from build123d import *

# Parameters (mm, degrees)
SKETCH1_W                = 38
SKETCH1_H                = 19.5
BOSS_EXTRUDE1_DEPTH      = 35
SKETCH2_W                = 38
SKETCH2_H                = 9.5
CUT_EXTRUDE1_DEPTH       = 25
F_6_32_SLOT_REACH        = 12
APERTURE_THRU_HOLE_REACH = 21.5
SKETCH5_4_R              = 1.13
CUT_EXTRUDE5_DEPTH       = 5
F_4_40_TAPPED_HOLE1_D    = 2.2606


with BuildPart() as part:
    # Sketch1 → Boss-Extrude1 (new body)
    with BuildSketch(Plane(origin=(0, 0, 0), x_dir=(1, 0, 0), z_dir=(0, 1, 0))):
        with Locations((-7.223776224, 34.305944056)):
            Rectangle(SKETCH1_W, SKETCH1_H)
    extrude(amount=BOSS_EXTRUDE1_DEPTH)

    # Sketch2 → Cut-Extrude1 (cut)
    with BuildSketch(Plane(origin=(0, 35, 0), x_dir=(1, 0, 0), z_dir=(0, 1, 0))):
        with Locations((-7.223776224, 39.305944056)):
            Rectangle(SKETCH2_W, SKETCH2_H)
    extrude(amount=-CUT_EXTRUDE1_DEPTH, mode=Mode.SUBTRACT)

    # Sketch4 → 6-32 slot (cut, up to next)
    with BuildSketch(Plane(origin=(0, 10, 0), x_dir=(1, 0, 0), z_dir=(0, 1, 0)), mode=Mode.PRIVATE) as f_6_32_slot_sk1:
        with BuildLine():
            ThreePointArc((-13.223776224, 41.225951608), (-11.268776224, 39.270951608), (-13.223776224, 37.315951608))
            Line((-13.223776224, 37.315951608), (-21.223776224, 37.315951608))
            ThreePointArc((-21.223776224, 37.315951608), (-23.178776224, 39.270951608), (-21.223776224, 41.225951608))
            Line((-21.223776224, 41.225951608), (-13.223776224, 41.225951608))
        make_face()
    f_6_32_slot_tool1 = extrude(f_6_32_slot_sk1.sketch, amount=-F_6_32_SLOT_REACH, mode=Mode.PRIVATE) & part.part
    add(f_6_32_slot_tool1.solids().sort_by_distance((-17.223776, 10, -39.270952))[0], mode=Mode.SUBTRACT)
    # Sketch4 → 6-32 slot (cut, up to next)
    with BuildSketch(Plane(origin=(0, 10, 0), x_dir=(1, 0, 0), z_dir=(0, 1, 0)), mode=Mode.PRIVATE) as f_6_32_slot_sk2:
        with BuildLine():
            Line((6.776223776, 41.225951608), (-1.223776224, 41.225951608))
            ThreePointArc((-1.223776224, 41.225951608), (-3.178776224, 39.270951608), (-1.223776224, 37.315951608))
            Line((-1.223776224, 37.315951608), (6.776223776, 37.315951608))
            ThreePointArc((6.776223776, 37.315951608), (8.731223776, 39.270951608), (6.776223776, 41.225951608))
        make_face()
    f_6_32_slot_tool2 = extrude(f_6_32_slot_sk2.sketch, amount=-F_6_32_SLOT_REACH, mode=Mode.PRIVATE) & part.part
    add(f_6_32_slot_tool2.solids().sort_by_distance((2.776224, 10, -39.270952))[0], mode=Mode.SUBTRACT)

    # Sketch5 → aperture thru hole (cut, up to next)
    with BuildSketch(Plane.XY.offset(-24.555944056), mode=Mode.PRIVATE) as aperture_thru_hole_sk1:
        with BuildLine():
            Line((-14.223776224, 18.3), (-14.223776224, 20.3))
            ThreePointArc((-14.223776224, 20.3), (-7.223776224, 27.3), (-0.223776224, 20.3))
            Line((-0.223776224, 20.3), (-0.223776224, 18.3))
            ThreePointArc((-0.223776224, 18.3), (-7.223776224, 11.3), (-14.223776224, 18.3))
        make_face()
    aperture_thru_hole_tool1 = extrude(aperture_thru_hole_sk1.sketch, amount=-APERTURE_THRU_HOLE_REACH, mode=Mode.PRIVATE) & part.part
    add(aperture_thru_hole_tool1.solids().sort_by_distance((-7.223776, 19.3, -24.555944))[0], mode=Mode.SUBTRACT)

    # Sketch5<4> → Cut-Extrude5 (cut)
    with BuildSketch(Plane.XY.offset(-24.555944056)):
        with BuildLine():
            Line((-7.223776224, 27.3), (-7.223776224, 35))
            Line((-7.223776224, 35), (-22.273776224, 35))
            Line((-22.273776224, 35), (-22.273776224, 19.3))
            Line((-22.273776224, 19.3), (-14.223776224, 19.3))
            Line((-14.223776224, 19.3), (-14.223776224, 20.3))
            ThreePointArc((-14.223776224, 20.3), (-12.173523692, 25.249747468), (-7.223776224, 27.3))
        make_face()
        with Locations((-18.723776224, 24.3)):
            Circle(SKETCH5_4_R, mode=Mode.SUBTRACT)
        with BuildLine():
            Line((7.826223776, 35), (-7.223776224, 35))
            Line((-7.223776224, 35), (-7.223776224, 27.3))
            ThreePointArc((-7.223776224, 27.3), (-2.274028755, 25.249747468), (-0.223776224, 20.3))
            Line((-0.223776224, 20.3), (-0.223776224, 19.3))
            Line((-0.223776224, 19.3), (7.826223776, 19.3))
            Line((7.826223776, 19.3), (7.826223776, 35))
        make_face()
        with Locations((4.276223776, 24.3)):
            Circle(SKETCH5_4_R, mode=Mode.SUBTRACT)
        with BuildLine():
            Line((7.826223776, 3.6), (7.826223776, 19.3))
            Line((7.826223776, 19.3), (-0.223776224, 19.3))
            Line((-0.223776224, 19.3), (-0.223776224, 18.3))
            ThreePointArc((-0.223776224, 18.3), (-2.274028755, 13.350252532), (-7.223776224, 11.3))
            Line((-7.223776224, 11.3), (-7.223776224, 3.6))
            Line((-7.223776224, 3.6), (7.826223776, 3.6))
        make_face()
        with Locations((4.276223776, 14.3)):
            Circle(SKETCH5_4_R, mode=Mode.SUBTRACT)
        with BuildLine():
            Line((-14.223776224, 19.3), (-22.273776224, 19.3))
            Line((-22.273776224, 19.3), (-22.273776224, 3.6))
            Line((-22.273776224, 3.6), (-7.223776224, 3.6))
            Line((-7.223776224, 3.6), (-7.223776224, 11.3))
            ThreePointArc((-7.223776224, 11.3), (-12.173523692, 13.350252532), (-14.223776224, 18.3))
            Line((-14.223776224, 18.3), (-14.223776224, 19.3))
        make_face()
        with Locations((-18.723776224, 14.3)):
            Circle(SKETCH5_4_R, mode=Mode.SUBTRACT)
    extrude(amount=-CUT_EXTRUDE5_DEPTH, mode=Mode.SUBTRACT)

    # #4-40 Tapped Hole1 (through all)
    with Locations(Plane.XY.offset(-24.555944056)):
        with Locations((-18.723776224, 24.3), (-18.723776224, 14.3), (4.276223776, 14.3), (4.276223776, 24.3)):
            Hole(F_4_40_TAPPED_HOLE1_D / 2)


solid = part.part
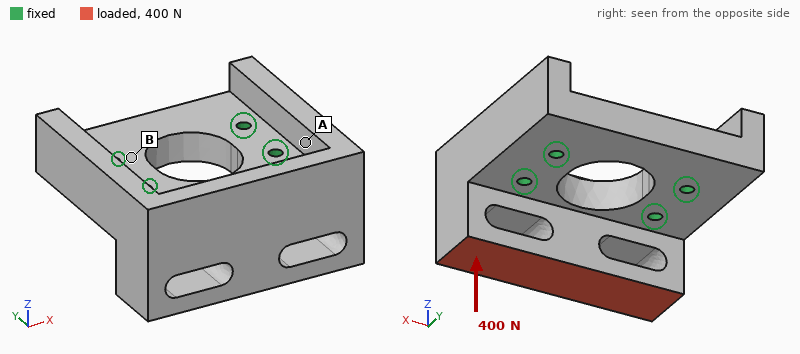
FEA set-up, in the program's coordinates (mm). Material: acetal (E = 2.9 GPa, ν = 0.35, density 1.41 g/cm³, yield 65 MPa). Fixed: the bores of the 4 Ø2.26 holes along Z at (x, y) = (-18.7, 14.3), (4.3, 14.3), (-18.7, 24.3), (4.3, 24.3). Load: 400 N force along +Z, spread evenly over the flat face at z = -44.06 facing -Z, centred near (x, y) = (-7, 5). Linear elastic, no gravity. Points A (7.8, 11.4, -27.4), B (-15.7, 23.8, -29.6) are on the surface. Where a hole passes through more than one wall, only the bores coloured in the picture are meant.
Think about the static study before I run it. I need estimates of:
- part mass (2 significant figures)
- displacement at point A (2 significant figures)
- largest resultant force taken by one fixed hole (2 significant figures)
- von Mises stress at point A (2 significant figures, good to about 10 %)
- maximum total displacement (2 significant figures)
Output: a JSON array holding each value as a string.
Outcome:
["15 g", "0.058 mm", "280 N", "5.7 MPa", "0.27 mm"]
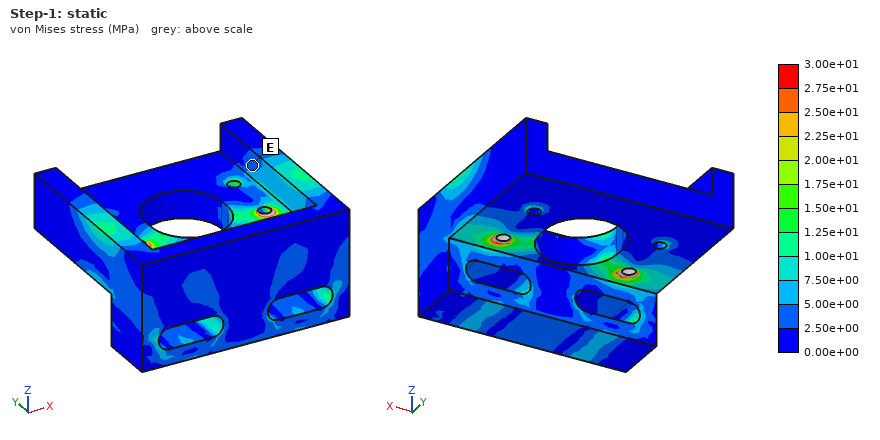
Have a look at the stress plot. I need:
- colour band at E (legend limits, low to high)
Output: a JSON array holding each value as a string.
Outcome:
["2.50e+00 to 5.00e+00 MPa"]
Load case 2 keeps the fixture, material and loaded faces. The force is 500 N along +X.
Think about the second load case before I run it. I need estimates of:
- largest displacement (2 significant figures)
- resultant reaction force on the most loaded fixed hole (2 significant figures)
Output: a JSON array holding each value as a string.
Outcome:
["0.20 mm", "390 N"]
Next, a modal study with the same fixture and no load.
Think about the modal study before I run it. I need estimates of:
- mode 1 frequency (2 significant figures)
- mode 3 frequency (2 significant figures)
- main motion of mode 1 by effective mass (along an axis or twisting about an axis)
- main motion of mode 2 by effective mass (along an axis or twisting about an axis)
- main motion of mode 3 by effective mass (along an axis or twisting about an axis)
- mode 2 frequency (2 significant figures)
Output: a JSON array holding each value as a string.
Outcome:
["2500 Hz", "6100 Hz", "along Z", "twisting about Y", "along X", "4000 Hz"]
